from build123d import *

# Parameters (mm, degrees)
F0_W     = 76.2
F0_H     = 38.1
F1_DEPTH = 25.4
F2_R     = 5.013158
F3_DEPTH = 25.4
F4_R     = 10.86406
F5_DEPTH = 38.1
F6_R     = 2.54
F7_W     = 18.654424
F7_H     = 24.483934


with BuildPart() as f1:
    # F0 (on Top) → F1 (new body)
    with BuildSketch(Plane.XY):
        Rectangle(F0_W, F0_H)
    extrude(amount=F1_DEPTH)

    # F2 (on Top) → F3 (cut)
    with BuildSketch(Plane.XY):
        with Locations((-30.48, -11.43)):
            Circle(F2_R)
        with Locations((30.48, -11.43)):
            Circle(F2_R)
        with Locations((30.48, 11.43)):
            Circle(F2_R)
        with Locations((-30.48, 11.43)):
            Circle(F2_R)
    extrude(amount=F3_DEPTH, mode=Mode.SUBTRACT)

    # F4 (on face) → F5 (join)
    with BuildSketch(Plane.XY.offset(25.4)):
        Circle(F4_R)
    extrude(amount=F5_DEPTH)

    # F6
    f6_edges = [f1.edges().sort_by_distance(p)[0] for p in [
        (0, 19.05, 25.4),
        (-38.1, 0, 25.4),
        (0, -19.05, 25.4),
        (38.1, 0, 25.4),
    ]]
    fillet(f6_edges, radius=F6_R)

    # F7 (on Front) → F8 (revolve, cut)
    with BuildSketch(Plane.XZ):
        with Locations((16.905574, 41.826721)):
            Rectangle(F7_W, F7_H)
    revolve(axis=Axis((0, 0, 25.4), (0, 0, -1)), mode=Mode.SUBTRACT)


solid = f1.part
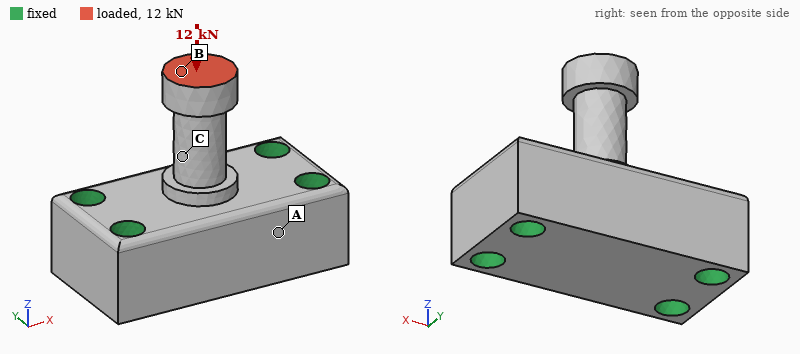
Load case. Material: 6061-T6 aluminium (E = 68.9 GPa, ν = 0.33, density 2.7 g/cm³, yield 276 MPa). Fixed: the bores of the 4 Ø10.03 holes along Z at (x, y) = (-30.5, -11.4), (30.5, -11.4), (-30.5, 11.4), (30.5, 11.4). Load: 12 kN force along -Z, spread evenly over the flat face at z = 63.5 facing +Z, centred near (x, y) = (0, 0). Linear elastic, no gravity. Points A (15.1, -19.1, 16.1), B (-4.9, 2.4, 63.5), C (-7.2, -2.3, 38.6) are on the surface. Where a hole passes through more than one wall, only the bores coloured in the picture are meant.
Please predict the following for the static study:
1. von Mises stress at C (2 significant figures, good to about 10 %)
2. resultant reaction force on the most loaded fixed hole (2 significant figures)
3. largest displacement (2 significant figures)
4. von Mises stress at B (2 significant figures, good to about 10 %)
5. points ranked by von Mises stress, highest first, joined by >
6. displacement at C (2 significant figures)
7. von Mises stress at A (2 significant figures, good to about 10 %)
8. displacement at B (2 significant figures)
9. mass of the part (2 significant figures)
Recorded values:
66 MPa
3.1 kN
44 µm
44 MPa
C > B > A
22 µm
14 MPa
42 µm
200 g
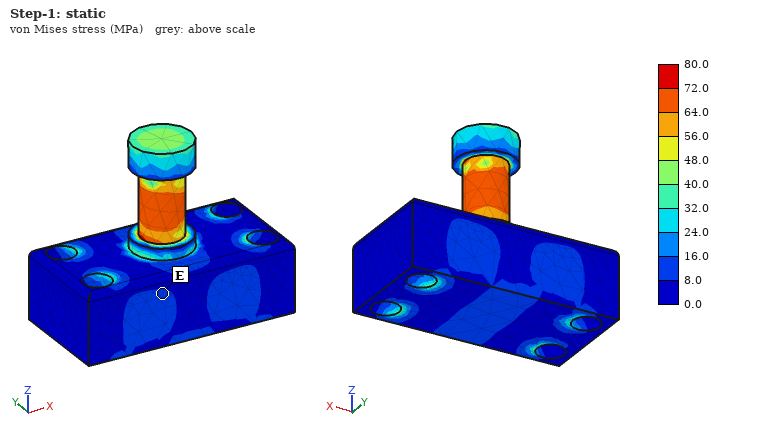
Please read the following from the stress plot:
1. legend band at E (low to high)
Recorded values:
8.0 to 16.0 MPa
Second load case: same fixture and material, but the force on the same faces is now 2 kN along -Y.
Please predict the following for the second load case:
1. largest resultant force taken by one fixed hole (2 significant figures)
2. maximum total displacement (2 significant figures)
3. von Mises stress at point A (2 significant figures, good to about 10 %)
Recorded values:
1.6 kN
0.24 mm
14 MPa
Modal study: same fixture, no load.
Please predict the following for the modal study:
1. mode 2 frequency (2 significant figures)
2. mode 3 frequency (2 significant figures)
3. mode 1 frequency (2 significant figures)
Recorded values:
5300 Hz
13 kHz
5100 Hz
